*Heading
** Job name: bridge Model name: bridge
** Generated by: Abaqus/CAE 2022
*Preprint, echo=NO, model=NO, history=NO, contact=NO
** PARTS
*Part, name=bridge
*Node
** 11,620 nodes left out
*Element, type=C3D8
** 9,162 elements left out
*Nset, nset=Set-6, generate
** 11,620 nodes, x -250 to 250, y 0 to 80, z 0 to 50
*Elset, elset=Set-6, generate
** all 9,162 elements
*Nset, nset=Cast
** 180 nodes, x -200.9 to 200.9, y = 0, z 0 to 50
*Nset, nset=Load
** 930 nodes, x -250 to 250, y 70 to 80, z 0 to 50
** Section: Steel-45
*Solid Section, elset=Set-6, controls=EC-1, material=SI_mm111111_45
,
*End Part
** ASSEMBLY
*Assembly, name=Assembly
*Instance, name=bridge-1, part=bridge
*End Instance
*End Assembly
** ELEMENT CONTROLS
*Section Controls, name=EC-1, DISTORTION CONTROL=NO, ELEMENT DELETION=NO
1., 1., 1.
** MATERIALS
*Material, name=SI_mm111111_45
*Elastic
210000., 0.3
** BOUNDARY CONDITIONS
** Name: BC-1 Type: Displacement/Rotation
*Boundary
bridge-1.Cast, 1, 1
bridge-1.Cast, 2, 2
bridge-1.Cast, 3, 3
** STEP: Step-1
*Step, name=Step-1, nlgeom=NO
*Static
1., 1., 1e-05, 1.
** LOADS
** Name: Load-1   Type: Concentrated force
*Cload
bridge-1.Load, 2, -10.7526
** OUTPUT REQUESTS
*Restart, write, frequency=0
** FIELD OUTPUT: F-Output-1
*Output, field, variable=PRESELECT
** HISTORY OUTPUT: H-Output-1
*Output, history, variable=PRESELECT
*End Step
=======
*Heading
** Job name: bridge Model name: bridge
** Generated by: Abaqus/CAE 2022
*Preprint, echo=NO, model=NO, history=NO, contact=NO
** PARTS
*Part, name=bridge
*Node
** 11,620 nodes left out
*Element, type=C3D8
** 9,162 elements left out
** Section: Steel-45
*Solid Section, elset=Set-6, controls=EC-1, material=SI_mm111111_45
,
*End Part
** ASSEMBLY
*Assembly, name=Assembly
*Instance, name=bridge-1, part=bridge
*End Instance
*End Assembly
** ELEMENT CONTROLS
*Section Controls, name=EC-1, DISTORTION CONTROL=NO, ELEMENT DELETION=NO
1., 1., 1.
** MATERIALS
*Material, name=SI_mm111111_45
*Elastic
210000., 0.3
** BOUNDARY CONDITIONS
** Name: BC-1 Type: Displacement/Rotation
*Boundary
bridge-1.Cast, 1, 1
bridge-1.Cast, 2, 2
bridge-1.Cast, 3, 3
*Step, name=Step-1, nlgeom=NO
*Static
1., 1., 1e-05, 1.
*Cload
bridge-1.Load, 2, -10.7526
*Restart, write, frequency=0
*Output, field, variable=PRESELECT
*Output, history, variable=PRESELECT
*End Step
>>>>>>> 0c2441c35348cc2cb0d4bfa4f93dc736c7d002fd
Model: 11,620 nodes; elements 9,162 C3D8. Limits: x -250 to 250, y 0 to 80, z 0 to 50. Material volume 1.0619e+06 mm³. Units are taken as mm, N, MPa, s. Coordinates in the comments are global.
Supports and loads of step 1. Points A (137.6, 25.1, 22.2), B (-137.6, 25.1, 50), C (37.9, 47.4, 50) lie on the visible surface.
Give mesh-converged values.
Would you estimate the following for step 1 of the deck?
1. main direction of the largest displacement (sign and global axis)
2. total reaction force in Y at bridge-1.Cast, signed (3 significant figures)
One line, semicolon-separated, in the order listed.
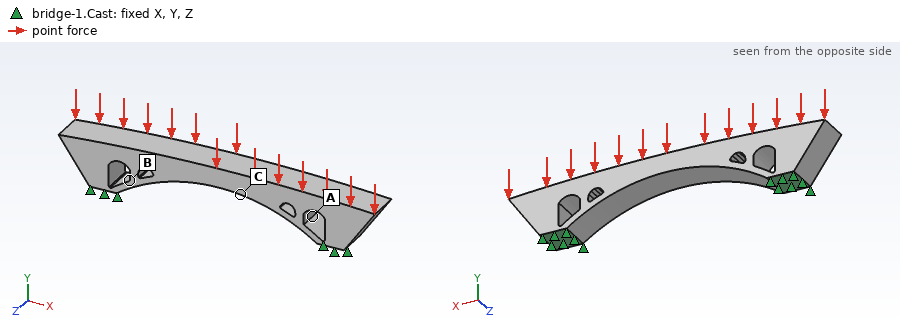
-Y; 10000 N
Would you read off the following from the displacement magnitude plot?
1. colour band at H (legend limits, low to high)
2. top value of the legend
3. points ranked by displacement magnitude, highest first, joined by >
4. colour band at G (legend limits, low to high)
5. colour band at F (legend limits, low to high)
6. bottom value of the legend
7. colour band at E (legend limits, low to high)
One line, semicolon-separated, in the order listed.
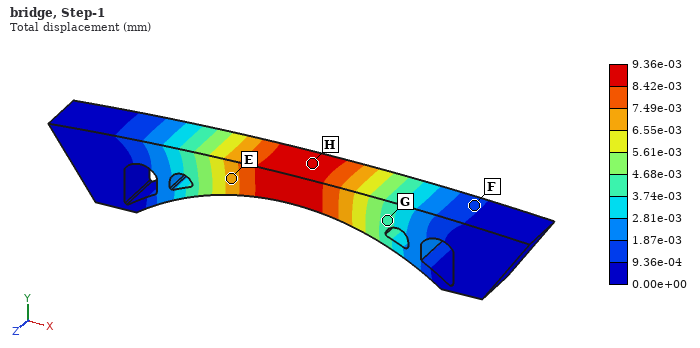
8.42e-03 to 9.36e-03 mm; 9.36e-03 mm; H > E > G > F; 3.74e-03 to 4.68e-03 mm; 9.36e-04 to 1.87e-03 mm; 0.00e+00 mm; 6.55e-03 to 7.49e-03 mm
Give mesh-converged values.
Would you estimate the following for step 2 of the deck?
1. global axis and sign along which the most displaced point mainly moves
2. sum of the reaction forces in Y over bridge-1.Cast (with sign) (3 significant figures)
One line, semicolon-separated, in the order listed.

-Y; 10000 N
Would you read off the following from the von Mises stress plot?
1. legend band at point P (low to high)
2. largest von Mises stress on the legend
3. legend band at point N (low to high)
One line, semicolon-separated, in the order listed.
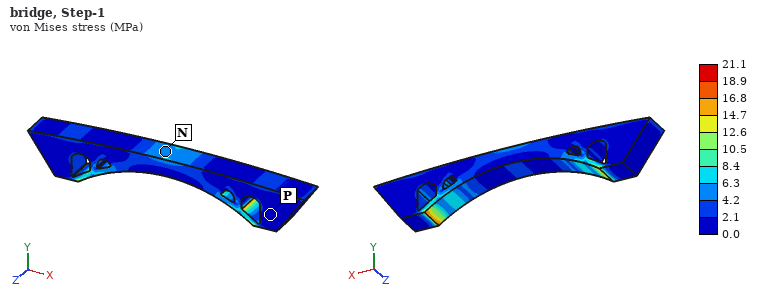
0.0 to 2.1 MPa; 21.1 MPa; 4.2 to 6.3 MPa
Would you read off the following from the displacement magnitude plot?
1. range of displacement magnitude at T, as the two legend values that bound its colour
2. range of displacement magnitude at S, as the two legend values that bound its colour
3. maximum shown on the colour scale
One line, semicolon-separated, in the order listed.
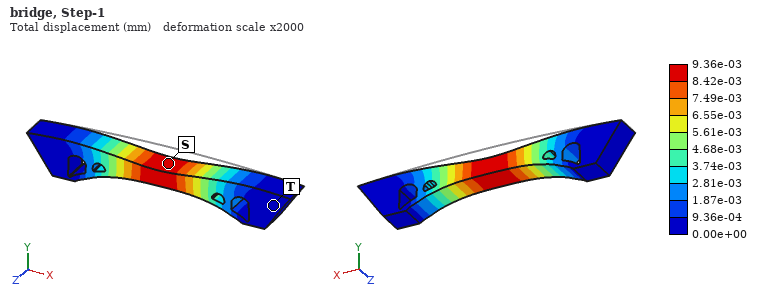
0.00e+00 to 9.36e-04 mm; 8.42e-03 to 9.36e-03 mm; 9.36e-03 mm
